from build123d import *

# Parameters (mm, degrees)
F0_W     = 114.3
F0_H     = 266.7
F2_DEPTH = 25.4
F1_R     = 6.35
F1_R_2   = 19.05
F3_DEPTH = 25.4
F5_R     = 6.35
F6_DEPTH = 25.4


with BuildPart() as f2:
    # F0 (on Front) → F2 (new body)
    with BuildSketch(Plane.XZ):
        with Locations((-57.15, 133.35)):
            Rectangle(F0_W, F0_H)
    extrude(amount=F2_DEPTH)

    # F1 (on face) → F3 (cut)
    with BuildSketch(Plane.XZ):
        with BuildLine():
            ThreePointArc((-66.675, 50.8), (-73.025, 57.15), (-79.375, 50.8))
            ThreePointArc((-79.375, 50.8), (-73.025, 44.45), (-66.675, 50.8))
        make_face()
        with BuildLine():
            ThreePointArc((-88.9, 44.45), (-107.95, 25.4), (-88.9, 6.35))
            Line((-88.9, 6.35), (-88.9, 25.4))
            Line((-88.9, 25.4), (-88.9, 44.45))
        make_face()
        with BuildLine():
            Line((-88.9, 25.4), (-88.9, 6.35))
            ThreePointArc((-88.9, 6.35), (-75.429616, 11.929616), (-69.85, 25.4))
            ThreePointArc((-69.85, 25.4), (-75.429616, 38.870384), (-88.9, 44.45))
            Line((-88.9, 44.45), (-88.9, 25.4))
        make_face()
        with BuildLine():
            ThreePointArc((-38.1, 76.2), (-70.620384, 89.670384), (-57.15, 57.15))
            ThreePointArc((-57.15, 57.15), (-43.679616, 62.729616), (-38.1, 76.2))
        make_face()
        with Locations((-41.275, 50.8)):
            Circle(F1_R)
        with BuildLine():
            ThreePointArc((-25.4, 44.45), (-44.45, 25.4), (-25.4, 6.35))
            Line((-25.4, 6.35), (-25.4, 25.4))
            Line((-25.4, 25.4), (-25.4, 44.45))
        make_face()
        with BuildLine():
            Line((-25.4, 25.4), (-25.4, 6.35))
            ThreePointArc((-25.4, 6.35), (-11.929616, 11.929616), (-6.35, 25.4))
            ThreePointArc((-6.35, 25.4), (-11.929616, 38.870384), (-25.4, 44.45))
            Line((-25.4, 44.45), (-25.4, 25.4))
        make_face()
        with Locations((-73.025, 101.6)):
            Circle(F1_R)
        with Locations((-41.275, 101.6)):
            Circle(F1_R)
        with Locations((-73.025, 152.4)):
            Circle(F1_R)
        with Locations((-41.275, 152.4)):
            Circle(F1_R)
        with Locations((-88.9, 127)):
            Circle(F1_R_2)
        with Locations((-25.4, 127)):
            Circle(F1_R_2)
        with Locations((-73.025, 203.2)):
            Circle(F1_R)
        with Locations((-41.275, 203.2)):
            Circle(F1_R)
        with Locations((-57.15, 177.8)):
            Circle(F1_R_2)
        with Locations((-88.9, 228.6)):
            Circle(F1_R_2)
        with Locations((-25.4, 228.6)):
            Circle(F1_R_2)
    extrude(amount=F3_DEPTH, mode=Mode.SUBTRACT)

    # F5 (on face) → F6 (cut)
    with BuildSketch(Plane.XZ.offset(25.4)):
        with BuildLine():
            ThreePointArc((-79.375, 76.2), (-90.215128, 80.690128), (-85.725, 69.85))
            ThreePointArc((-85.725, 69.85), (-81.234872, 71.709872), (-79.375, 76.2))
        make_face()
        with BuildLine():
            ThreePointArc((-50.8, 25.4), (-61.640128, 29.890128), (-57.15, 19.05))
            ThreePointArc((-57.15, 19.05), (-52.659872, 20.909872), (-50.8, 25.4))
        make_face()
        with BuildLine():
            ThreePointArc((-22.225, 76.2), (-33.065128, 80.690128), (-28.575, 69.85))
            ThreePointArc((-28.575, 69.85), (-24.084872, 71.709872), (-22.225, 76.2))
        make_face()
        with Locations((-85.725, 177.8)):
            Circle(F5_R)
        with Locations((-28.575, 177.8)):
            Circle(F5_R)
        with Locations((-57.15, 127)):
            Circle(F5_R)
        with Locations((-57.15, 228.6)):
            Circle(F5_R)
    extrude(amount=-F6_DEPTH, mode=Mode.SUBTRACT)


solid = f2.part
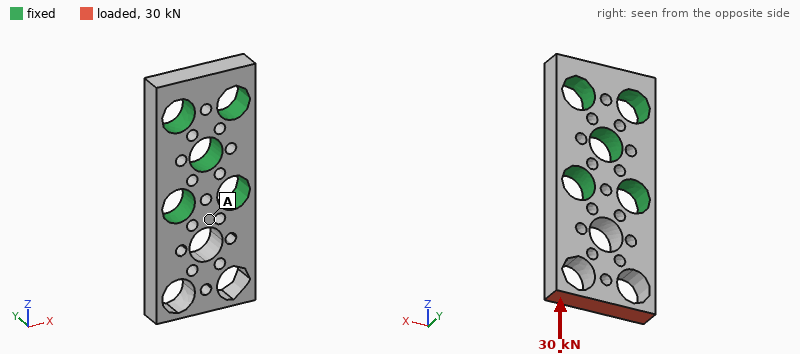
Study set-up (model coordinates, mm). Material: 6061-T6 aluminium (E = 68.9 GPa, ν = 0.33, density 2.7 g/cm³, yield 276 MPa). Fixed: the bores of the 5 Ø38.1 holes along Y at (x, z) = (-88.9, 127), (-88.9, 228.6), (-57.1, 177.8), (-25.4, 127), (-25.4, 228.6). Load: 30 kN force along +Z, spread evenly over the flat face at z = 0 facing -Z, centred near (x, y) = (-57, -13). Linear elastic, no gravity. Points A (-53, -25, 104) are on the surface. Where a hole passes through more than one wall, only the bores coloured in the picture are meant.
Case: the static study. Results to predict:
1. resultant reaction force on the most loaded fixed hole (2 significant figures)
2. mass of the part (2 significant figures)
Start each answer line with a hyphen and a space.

- 15 kN
- 1.3 kg
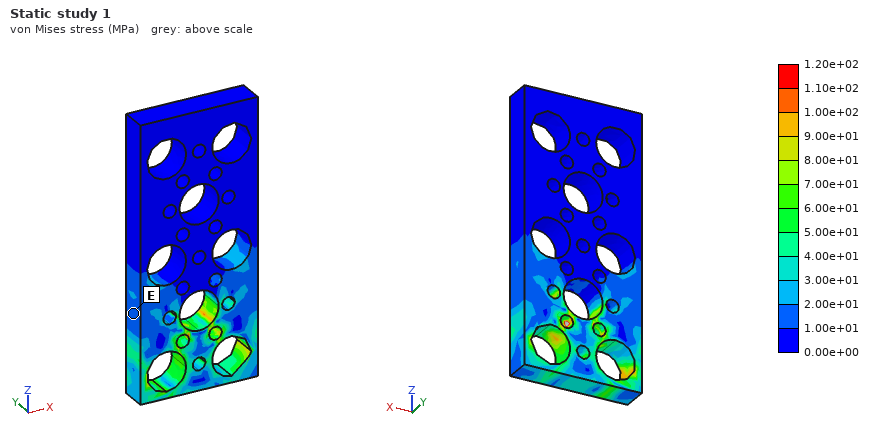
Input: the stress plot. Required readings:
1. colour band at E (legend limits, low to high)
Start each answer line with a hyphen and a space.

- 1.00e+01 to 2.00e+01 MPa
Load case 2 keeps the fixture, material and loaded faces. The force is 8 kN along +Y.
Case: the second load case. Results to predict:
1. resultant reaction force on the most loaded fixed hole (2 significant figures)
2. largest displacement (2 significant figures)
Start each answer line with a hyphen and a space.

- 4.0 kN
- 0.69 mm
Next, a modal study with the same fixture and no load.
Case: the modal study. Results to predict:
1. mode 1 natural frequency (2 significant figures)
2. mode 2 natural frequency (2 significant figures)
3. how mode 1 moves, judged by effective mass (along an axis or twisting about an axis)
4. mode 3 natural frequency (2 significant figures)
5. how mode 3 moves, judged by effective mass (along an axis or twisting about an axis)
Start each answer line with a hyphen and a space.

- 1600 Hz
- 3000 Hz
- along Y
- 3600 Hz
- along X
